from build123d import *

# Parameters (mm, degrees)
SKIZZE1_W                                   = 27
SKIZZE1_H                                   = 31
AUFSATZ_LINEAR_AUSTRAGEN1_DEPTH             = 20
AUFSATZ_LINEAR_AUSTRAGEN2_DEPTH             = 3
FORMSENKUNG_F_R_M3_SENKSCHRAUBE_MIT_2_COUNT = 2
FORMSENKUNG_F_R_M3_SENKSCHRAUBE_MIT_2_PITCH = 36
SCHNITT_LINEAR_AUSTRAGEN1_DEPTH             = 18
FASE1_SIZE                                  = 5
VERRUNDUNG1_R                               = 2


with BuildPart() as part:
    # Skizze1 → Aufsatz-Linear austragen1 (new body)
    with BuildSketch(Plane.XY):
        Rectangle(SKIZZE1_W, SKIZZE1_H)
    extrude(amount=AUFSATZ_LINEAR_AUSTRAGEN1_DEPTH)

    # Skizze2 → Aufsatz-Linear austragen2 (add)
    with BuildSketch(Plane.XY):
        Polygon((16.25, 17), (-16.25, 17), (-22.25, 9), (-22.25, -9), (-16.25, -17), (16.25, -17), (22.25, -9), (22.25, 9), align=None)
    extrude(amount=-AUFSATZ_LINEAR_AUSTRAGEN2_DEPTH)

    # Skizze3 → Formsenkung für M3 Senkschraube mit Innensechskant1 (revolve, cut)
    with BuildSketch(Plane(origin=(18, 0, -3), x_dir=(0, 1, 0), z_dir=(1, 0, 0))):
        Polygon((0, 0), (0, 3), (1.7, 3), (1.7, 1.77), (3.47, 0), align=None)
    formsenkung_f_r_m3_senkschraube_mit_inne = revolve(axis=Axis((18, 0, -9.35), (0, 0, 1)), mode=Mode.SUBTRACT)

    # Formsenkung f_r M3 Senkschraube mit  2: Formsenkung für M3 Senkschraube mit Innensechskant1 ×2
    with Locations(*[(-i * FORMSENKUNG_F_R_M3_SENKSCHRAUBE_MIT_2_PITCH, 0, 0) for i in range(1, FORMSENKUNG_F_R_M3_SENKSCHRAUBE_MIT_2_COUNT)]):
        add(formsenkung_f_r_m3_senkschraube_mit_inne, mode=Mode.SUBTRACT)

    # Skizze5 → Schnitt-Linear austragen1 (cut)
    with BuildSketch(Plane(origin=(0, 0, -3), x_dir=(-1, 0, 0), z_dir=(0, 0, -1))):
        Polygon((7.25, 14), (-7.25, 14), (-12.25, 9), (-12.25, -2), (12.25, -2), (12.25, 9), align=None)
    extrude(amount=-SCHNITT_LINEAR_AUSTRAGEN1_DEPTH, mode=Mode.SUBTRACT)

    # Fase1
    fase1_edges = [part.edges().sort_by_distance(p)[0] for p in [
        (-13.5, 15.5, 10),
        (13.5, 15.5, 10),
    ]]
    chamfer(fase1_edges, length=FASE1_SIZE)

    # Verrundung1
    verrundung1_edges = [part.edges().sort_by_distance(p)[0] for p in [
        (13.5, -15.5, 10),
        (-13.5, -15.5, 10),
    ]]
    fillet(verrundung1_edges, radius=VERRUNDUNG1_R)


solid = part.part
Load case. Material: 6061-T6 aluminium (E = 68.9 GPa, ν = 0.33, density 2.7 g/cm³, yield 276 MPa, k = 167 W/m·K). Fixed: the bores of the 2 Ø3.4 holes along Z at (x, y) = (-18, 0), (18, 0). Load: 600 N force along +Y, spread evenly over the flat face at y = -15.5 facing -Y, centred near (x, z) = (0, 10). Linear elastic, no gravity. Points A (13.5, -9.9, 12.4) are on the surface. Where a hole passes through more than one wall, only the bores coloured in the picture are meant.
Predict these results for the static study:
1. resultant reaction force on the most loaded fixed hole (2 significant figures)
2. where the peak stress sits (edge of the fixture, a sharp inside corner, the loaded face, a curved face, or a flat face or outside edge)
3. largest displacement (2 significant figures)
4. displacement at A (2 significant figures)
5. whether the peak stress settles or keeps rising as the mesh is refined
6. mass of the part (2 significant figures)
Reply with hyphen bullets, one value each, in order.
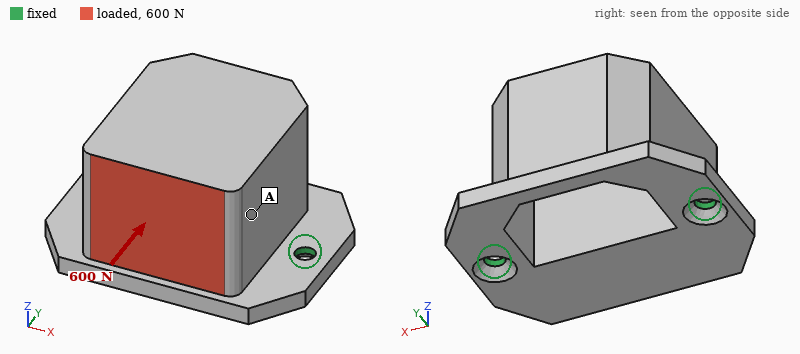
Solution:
- 310 N
- edge of the fixture
- 0.22 mm
- 0.14 mm
- keeps rising
- 37 g
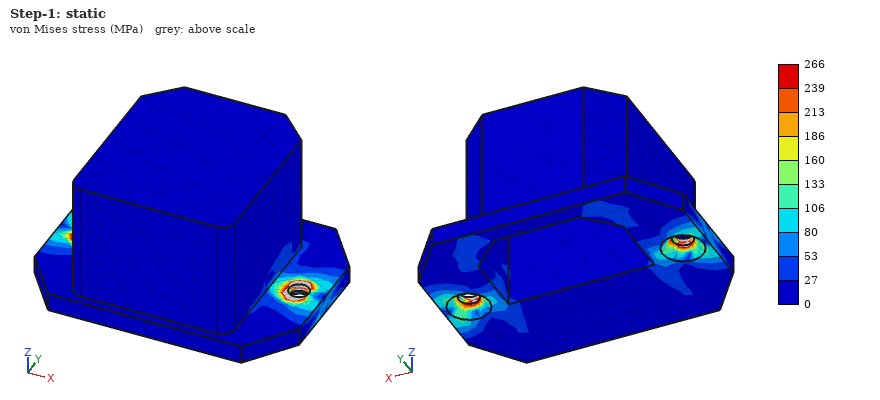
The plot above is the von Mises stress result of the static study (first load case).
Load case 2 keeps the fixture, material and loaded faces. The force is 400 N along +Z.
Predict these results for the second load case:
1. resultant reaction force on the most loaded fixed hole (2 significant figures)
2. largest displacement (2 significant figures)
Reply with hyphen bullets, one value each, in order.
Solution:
- 200 N
- 0.20 mm
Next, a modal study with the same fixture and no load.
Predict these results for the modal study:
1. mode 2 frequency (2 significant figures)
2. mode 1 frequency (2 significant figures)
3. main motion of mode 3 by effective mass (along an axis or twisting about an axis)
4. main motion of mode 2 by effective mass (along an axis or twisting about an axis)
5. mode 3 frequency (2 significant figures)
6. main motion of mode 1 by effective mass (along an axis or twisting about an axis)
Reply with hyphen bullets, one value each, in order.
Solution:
- 6500 Hz
- 1500 Hz
- along Z
- along X
- 6800 Hz
- along Y
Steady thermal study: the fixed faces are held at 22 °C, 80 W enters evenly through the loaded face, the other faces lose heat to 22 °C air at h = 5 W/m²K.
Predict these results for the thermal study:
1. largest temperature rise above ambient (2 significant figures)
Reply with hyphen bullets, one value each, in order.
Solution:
- 71 K
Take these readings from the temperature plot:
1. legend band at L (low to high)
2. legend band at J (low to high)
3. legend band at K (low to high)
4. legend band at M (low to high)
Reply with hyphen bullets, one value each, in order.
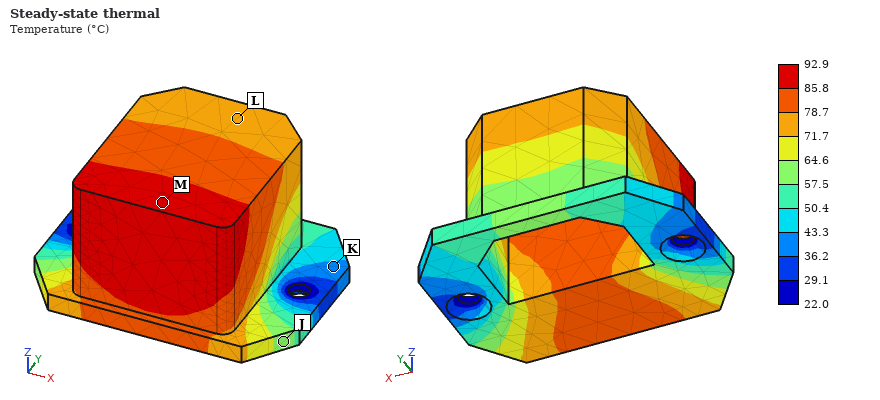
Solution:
- 71.7 to 78.7 °C
- 57.5 to 64.6 °C
- 36.2 to 43.3 °C
- 85.8 to 92.9 °C
